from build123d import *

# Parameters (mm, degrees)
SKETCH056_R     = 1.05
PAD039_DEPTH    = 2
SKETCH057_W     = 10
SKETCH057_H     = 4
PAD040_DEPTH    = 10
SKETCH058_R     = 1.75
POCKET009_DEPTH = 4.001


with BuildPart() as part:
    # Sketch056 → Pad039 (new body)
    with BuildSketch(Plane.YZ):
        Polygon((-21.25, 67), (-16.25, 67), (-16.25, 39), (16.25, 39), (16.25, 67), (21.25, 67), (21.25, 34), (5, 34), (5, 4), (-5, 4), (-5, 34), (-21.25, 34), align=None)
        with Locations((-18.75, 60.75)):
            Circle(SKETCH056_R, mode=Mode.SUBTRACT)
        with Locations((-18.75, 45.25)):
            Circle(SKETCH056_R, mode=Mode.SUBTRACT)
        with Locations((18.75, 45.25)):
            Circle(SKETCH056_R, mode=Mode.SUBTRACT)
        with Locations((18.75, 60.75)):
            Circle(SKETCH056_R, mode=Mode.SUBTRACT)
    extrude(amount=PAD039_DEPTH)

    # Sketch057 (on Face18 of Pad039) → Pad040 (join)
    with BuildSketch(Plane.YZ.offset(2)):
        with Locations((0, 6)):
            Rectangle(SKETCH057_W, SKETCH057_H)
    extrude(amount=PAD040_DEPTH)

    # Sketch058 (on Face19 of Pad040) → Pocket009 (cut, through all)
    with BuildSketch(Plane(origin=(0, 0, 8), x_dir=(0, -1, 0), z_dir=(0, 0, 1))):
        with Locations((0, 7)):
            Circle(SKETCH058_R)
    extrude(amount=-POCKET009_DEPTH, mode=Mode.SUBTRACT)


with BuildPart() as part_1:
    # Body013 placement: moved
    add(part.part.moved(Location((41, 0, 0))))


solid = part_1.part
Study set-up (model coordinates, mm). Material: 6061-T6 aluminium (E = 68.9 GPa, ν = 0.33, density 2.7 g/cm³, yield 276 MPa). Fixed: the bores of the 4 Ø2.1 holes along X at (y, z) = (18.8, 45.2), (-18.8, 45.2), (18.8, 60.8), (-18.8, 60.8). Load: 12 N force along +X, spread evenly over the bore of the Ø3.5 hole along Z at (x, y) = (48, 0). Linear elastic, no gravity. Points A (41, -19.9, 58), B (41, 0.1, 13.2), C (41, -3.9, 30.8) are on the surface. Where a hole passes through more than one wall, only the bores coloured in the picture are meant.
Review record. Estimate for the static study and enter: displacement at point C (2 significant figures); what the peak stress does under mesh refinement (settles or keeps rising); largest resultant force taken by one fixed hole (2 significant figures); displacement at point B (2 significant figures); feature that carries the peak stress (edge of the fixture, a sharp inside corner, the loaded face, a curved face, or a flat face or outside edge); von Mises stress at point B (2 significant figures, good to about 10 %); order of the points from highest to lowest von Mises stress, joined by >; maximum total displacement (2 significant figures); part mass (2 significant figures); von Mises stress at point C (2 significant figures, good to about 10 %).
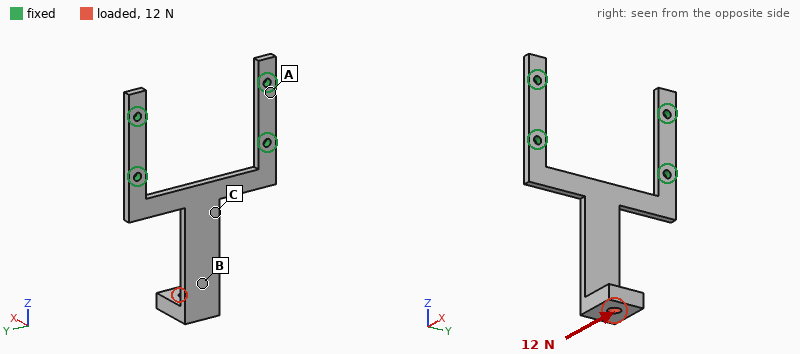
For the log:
0.16 mm
keeps rising
6.2 N
0.58 mm
edge of the fixture
13 MPa
C > B > A
0.90 mm
5.2 g
46 MPa
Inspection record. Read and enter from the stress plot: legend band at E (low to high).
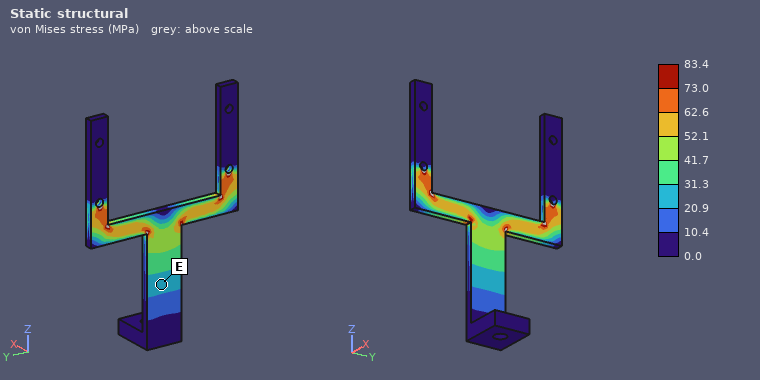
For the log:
20.9 to 31.3 MPa
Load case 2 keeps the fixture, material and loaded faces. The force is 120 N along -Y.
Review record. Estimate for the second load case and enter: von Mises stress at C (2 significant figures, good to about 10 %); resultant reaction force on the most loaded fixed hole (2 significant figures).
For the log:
110 MPa
140 N
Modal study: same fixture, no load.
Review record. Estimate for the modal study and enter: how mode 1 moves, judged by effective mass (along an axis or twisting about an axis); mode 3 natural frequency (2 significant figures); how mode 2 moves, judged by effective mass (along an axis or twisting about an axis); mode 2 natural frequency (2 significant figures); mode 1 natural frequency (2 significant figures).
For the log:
along X
3000 Hz
along Y
2300 Hz
480 Hz
